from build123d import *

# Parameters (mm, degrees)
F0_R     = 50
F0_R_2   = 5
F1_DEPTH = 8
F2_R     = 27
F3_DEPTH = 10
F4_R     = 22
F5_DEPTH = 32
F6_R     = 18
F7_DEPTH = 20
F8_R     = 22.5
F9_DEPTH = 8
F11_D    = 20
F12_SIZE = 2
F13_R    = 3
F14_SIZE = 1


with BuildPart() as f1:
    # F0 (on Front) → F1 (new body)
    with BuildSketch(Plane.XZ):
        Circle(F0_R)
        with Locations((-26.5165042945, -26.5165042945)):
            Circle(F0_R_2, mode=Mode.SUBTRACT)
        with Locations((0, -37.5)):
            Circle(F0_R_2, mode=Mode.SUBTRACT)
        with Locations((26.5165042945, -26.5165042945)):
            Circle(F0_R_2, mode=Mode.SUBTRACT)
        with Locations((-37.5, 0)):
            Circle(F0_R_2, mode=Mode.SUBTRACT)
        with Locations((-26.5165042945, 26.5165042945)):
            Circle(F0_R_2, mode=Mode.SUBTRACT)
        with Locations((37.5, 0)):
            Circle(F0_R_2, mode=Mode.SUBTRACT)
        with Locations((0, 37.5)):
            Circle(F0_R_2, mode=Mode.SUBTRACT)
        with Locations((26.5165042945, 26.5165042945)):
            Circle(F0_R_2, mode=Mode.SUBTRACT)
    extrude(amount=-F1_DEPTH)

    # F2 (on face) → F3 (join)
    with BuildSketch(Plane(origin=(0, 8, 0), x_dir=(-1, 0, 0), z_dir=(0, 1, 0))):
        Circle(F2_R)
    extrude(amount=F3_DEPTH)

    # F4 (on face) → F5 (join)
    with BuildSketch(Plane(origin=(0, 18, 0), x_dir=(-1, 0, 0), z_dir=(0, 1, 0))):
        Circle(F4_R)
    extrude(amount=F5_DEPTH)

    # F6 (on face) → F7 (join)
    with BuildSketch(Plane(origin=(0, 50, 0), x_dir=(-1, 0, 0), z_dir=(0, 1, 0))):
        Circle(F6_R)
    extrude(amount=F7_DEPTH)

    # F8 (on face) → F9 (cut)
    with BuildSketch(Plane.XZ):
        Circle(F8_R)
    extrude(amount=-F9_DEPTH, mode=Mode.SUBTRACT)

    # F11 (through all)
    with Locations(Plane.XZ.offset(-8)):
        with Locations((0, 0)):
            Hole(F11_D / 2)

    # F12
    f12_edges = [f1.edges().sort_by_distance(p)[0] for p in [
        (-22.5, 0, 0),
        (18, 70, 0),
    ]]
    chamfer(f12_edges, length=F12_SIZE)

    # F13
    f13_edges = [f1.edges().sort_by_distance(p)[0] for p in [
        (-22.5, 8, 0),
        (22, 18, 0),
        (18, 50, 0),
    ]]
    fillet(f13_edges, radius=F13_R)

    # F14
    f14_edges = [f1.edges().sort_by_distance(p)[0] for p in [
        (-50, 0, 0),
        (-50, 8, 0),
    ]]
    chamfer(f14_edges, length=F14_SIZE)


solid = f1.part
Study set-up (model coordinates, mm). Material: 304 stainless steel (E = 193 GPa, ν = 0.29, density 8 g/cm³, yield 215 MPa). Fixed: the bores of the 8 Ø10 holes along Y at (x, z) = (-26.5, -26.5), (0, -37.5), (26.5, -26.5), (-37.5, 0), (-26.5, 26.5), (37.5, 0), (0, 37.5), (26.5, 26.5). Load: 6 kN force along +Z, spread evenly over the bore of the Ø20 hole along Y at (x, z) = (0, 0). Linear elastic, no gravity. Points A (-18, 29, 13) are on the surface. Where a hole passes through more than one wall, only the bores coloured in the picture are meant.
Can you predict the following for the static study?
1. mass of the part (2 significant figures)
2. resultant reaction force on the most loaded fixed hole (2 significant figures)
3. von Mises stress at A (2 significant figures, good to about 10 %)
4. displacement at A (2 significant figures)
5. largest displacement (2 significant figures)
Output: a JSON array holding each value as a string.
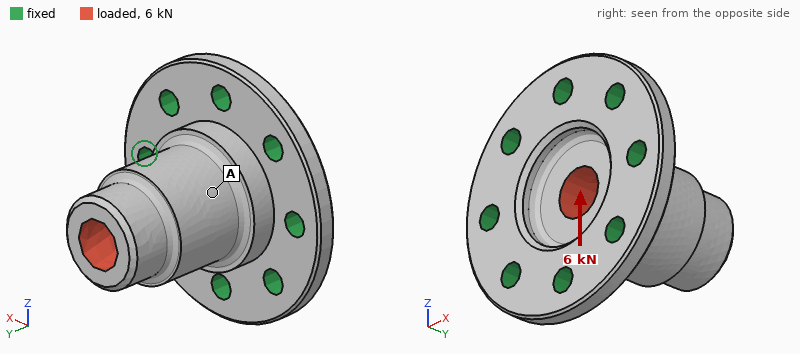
["940 g", "2.2 kN", "8.0 MPa", "4.7 µm", "14 µm"]
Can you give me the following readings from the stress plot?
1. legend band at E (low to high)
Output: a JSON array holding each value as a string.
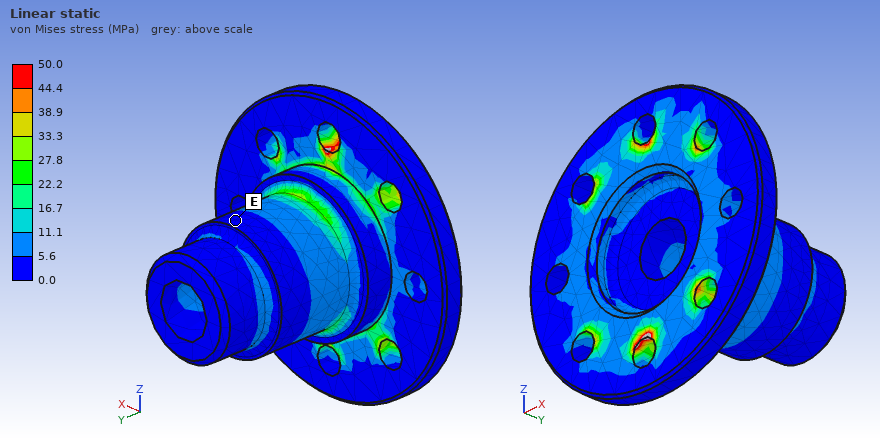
["0.0 to 5.6 MPa"]
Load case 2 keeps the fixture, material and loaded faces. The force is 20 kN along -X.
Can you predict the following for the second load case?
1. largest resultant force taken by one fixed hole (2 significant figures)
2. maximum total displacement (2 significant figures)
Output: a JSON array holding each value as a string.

["7.5 kN", "45 µm"]
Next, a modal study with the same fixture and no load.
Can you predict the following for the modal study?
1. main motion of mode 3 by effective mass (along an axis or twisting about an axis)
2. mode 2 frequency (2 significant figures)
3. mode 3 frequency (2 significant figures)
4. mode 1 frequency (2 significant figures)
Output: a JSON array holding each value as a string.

["along Y", "6100 Hz", "12 kHz", "6100 Hz"]
